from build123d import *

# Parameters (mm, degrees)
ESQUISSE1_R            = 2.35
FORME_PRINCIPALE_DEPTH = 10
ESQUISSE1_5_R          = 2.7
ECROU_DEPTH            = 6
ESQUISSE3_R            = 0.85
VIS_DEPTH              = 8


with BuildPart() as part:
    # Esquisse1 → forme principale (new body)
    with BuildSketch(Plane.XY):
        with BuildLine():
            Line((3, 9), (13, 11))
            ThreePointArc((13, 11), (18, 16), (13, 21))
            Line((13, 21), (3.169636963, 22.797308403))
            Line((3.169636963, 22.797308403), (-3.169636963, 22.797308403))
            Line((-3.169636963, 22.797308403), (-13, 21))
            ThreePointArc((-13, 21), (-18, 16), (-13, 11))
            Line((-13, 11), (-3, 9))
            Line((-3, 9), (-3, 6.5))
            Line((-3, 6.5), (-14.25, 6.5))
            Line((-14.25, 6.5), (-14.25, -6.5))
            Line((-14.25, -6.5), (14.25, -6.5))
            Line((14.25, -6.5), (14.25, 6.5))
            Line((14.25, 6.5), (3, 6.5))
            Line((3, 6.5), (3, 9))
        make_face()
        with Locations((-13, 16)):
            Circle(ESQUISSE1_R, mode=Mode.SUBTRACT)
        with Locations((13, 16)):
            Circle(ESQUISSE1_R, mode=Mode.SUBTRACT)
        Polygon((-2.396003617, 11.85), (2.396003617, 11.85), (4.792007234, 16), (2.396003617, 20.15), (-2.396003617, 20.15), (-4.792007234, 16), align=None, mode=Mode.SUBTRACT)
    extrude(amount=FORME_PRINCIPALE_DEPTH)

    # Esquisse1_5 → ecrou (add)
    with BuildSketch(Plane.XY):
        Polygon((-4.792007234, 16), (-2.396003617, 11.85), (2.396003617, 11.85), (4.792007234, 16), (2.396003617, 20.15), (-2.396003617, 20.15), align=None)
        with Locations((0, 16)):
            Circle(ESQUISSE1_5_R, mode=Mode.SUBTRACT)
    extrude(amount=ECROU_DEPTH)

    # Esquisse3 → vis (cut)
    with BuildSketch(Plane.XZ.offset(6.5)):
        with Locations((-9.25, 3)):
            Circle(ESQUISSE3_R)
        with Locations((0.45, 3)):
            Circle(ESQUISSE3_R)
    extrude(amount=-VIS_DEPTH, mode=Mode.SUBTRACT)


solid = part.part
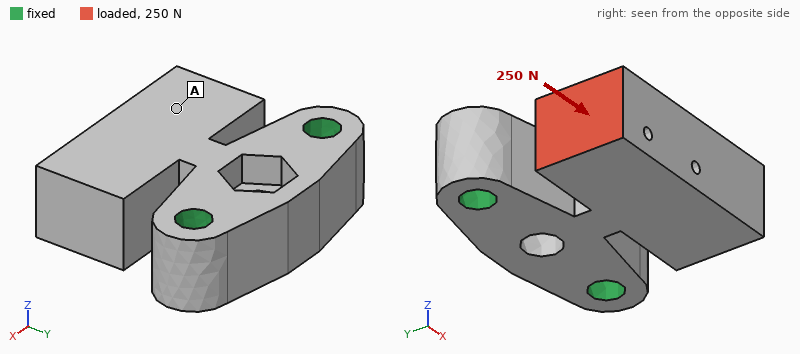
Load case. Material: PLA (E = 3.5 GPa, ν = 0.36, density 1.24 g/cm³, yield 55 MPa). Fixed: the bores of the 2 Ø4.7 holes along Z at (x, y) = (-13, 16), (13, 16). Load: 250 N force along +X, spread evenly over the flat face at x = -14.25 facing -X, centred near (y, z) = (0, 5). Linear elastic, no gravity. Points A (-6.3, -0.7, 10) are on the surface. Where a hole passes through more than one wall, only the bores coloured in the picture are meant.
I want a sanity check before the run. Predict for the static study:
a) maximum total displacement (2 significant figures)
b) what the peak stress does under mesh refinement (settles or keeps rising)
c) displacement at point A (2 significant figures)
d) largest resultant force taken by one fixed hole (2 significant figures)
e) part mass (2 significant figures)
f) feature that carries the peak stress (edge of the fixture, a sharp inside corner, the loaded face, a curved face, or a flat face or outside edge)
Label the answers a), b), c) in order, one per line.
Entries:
a) 0.51 mm
b) keeps rising
c) 0.28 mm
d) 240 N
e) 8.8 g
f) a sharp inside corner
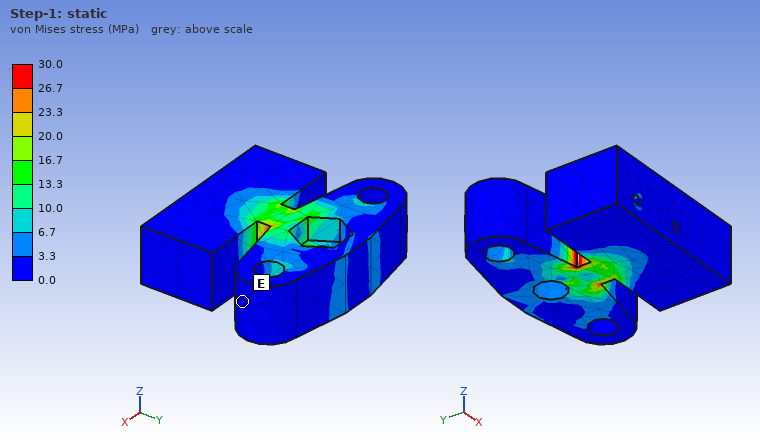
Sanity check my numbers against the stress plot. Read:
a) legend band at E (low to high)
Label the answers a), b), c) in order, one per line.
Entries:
a) 0.0 to 3.3 MPa
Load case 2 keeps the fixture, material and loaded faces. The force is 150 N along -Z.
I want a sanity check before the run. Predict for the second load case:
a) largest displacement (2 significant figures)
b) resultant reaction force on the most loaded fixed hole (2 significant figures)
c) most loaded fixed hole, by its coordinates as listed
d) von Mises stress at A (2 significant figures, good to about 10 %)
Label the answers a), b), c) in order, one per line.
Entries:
a) 0.55 mm
b) 170 N
c) (-13, 16)
d) 4.9 MPa
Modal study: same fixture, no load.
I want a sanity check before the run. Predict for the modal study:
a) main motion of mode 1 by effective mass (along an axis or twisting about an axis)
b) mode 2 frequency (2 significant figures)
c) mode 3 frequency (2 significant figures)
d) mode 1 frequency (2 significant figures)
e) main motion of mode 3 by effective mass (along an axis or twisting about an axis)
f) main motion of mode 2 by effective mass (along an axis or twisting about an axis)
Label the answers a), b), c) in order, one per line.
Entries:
a) along X
b) 2000 Hz
c) 3000 Hz
d) 1800 Hz
e) twisting about Y
f) along Z
